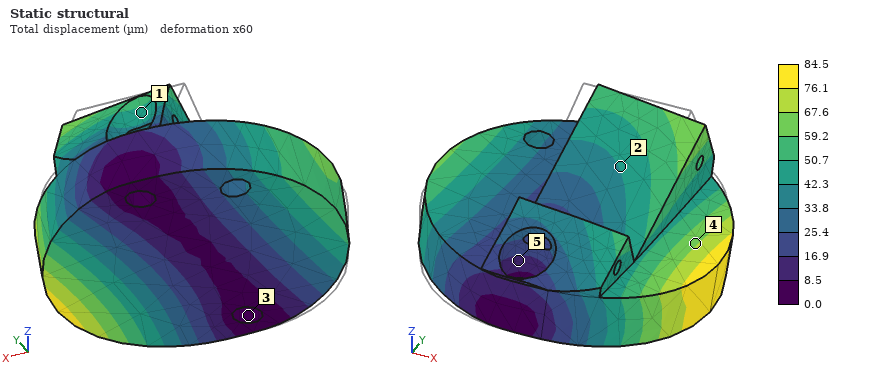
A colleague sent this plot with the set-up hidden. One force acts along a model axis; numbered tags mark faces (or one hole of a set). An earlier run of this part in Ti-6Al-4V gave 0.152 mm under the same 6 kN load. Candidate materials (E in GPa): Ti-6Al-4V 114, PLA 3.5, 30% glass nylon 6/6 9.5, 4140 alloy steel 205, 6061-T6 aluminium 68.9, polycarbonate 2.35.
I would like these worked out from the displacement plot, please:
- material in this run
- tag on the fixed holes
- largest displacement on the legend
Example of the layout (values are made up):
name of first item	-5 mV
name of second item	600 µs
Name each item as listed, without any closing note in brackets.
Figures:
material in this run	4140 alloy steel
tag on the fixed holes	3
largest displacement on the legend	84.5 µm
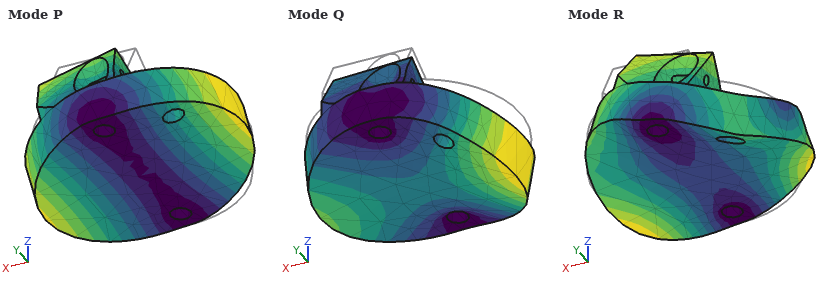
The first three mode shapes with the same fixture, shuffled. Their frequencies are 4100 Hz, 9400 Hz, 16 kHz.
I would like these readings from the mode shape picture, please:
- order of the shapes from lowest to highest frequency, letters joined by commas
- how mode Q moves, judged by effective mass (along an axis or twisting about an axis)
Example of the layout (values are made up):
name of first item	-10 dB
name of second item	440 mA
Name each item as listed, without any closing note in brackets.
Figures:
order of the shapes from lowest to highest frequency, letters joined by commas	P, Q, R
how mode Q moves, judged by effective mass	along Z
